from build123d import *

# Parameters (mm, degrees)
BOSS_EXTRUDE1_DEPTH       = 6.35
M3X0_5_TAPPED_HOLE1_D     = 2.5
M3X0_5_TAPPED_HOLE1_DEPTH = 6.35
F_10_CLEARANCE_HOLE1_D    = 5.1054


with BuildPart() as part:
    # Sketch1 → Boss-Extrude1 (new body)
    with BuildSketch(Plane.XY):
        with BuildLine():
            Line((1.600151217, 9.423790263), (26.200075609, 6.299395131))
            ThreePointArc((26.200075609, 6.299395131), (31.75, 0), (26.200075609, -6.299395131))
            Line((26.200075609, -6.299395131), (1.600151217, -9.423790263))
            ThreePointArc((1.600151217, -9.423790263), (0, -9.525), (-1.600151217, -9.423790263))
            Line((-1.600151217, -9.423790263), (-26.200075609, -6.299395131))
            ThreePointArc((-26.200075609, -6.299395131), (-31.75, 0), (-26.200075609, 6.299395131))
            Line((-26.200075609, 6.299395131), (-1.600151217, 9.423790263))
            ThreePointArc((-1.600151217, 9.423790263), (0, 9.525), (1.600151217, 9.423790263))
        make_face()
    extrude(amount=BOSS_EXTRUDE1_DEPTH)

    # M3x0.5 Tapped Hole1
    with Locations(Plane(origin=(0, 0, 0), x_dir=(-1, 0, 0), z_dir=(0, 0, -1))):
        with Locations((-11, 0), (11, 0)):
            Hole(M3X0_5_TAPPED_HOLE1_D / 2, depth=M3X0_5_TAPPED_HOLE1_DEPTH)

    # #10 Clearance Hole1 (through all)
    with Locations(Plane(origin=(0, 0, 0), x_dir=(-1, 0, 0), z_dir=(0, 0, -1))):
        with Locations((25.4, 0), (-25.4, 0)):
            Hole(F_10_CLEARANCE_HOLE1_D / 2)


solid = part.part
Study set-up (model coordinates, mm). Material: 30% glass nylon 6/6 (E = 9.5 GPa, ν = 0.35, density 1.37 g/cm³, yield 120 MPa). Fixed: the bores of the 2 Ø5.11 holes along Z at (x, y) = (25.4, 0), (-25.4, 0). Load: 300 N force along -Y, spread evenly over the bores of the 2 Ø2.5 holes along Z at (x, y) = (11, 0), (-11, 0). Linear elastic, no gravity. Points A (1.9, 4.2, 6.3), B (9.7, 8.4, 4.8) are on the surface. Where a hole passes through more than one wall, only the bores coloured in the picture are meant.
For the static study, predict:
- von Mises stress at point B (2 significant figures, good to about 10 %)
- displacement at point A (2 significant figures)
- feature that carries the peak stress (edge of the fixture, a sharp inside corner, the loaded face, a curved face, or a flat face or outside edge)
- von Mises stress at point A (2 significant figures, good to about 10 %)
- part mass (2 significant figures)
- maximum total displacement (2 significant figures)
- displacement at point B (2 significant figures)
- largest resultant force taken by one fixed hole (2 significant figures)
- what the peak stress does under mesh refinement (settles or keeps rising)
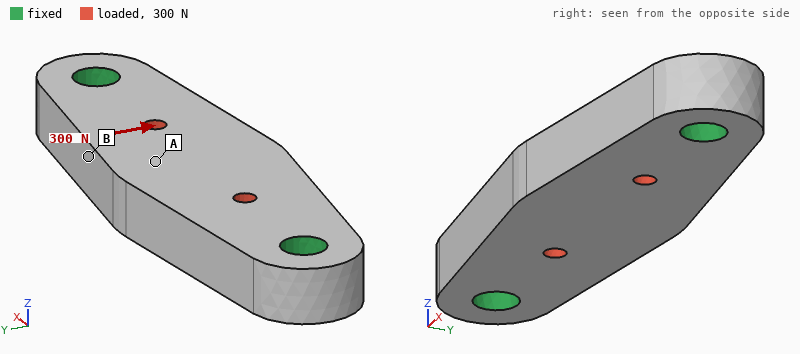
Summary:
4.4 MPa
17 µm
edge of the fixture
1.5 MPa
7.7 g
17 µm
15 µm
150 N
keeps rising
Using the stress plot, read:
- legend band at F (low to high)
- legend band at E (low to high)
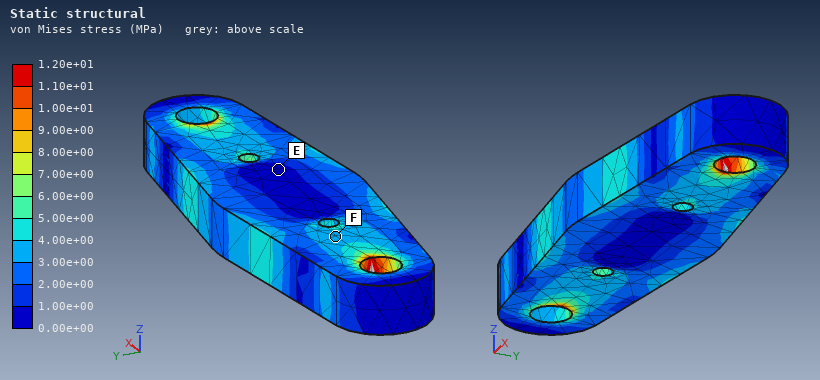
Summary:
3.00e+00 to 4.00e+00 MPa
0.00e+00 to 1.00e+00 MPa
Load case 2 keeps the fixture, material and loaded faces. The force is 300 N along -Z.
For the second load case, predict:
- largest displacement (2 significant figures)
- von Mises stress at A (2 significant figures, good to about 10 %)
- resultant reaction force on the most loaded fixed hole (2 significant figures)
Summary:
41 µm
4.8 MPa
150 N
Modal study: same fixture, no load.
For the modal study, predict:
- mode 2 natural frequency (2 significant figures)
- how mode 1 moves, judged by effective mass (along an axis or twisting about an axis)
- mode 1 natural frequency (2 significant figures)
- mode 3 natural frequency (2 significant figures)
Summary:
9100 Hz
along Z
6100 Hz
9500 Hz
